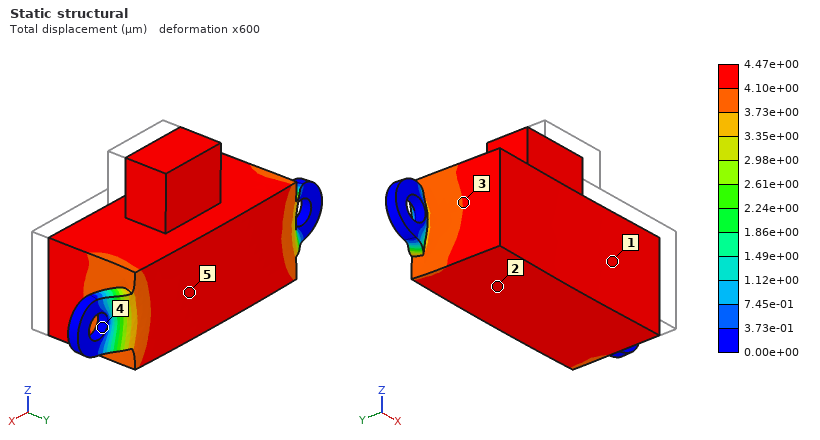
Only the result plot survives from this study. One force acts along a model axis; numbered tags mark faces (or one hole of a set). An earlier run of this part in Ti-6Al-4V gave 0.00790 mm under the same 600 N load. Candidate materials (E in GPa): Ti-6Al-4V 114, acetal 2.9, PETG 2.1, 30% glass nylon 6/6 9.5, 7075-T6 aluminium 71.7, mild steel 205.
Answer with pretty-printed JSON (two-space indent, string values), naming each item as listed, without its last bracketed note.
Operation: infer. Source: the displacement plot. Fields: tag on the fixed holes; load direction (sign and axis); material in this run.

{
  "tag on the fixed holes": "4",
  "load direction": "+Y",
  "material in this run": "mild steel"
}
